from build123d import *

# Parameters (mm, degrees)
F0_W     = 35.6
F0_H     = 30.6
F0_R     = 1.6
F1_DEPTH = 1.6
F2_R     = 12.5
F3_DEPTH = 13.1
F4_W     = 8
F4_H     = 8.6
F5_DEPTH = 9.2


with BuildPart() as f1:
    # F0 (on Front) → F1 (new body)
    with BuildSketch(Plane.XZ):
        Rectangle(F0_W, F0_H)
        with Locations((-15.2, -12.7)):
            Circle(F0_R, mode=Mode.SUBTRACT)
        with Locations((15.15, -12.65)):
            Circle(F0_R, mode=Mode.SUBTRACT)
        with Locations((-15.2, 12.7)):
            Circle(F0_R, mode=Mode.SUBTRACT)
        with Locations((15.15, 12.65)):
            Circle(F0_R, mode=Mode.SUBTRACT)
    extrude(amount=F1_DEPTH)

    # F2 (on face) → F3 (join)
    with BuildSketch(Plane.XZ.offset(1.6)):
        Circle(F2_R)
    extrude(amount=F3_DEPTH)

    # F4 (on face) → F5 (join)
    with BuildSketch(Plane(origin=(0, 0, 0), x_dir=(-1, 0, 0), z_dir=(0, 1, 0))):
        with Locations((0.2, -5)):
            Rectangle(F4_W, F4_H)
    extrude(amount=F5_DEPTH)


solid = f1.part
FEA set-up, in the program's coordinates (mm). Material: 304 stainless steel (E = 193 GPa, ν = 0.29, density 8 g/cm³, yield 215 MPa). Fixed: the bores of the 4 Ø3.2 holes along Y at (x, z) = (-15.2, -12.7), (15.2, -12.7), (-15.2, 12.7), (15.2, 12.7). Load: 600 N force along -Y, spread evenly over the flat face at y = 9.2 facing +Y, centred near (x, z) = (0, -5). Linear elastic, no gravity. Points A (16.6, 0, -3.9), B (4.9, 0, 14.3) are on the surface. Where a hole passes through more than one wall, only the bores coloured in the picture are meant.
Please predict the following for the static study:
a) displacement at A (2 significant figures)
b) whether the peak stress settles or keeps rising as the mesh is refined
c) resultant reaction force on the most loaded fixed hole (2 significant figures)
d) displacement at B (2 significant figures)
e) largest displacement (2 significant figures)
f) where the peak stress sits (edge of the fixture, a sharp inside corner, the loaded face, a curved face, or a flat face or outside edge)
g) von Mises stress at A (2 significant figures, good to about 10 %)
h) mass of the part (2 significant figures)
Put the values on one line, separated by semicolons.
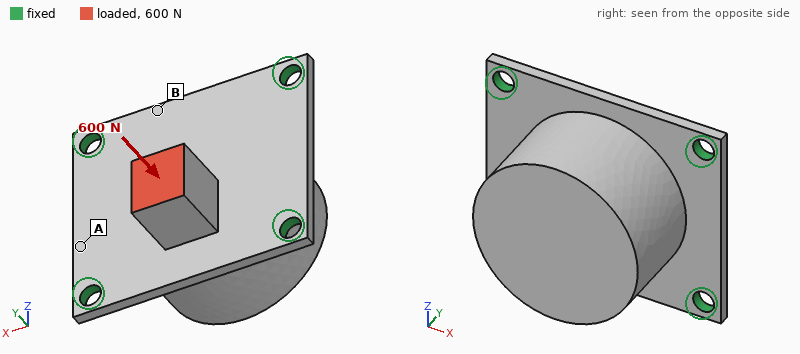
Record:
5.7 µm; keeps rising; 230 N; 2.5 µm; 14 µm; edge of the fixture; 35 MPa; 70 g
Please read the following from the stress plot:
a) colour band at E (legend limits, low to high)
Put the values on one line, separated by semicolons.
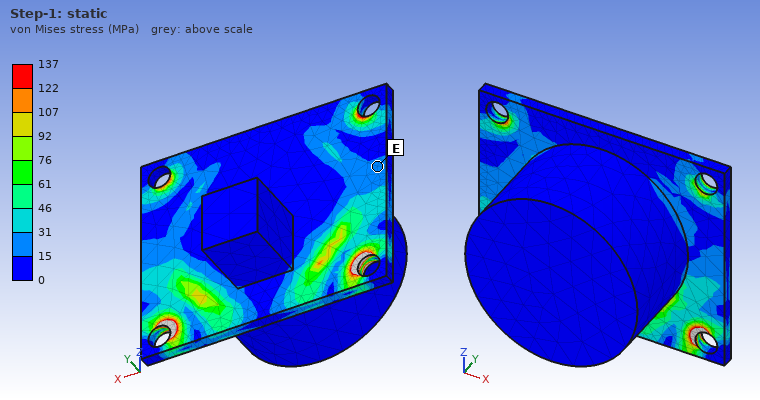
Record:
15 to 31 MPa
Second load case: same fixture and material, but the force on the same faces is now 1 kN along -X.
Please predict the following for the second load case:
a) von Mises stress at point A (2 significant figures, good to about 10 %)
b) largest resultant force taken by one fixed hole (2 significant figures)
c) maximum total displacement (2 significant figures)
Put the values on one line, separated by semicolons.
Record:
38 MPa; 390 N; 21 µm
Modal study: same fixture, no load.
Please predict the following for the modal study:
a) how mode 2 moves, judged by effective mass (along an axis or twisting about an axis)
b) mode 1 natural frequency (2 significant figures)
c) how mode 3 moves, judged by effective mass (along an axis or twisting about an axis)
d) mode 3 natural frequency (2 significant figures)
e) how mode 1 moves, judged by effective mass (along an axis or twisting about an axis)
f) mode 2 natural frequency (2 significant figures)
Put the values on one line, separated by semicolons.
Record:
along Z; 5300 Hz; along X; 6700 Hz; along Y; 5600 Hz
